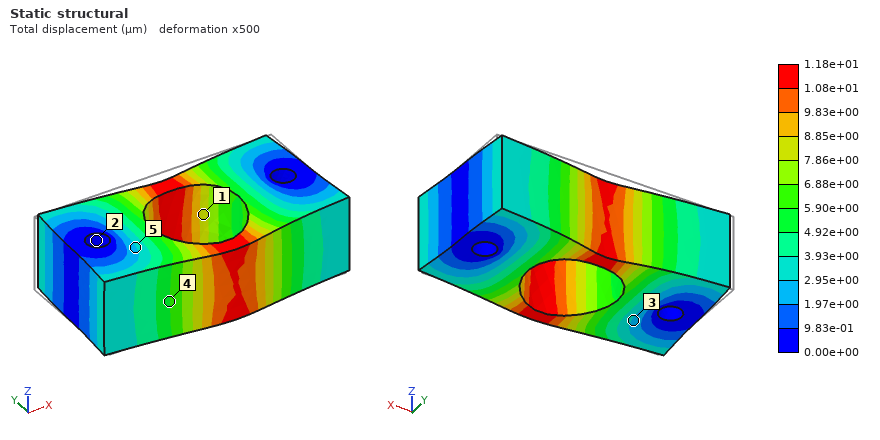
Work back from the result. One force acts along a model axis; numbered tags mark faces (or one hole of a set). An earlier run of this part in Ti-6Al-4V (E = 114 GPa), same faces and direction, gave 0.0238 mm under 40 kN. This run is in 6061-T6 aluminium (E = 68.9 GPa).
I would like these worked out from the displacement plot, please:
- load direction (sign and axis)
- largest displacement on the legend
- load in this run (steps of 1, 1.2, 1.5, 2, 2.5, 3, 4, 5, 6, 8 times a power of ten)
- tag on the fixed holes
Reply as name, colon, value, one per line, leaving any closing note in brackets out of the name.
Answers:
load direction: -Y
largest displacement on the legend: 1.18e+01 µm
load in this run: 12 kN
tag on the fixed holes: 2
